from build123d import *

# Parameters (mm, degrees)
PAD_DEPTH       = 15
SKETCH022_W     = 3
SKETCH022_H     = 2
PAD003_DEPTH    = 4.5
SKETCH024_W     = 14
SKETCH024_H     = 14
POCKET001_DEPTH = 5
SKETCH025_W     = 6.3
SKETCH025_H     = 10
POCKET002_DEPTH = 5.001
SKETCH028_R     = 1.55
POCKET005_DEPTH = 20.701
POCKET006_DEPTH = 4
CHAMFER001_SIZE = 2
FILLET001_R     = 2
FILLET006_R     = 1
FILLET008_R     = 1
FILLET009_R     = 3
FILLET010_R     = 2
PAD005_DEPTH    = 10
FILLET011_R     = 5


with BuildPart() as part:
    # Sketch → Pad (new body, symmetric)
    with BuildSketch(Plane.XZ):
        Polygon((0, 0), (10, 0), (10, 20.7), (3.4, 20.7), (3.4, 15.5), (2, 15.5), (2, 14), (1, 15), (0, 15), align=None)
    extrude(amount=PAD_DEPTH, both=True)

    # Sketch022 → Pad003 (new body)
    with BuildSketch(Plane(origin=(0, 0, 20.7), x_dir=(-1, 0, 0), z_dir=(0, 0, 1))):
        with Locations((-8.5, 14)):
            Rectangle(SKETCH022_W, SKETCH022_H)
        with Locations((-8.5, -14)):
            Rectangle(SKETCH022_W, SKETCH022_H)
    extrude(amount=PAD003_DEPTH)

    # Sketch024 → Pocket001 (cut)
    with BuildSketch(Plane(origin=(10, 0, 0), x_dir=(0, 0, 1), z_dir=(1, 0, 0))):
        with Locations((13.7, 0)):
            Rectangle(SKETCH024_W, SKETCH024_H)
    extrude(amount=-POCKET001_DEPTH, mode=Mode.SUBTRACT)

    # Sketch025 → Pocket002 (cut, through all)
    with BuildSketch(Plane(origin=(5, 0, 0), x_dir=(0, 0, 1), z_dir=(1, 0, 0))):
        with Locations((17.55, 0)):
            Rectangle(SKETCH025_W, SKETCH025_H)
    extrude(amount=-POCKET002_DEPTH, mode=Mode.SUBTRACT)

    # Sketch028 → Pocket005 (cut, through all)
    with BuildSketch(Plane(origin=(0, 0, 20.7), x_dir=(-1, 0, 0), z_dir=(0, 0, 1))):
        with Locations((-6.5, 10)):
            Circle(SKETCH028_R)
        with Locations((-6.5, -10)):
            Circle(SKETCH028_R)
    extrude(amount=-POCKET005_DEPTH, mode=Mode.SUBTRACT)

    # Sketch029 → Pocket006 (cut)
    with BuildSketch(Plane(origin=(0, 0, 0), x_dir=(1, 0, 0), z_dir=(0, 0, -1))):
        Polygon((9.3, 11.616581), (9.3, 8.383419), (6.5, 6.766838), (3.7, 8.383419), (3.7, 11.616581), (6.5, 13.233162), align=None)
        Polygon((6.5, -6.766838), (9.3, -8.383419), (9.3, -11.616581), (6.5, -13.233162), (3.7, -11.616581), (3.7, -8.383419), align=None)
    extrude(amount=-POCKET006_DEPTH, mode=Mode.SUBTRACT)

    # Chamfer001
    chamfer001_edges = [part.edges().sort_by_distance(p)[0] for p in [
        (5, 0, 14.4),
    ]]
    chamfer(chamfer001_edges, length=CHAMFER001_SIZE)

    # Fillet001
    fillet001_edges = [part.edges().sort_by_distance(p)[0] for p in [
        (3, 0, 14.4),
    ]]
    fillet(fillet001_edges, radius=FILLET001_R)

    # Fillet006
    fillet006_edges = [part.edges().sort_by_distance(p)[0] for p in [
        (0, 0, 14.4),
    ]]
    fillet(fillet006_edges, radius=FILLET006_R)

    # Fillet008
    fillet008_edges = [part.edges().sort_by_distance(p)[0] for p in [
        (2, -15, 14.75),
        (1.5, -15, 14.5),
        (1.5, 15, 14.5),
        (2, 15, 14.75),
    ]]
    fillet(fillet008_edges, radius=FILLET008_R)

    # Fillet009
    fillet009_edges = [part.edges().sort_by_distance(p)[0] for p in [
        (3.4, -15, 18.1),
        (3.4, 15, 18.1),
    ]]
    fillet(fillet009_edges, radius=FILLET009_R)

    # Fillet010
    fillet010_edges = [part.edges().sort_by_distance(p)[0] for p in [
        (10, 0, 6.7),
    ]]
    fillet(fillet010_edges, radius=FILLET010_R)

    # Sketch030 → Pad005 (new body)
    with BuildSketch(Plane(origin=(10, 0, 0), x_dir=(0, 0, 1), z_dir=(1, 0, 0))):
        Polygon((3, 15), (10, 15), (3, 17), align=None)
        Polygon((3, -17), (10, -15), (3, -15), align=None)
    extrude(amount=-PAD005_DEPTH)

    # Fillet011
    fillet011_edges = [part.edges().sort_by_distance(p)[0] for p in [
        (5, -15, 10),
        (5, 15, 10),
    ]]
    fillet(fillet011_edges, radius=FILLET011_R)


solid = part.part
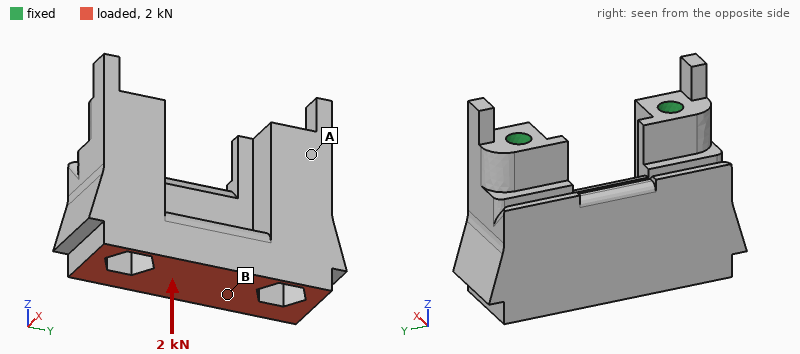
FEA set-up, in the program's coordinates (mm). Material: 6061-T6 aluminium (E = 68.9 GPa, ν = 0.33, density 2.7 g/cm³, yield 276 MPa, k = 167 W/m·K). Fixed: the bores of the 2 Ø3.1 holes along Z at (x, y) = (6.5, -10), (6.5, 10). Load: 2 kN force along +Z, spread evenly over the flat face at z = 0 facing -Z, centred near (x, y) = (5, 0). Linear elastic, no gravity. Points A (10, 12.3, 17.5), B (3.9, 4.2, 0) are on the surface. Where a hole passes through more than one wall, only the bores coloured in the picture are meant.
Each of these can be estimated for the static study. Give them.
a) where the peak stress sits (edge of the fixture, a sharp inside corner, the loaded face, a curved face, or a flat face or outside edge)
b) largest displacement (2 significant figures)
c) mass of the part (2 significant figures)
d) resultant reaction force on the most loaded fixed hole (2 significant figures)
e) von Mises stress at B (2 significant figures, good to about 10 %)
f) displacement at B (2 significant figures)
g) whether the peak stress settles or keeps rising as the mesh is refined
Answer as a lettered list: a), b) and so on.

a) edge of the fixture
b) 3.8 µm
c) 11 g
d) 1.0 kN
e) 8.7 MPa
f) 2.6 µm
g) keeps rising
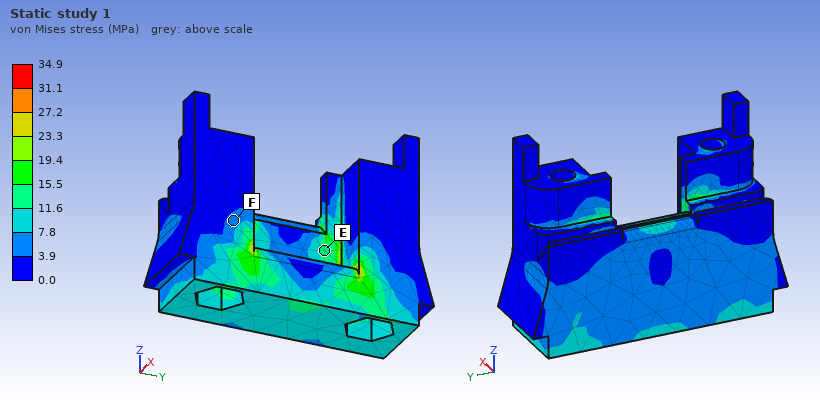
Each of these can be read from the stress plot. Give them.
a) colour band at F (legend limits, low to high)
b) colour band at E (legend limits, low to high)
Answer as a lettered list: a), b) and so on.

a) 3.9 to 7.8 MPa
b) 11.6 to 15.5 MPa
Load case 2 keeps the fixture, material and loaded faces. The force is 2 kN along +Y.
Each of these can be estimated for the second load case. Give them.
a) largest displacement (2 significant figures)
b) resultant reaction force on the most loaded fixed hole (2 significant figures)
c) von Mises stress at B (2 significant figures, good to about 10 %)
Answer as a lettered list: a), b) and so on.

a) 5.9 µm
b) 1.1 kN
c) 16 MPa
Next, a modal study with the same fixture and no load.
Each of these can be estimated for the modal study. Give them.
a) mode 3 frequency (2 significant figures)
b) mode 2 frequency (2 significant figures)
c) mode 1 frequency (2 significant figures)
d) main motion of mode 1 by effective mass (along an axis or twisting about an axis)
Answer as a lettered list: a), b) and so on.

a) 50 kHz
b) 50 kHz
c) 43 kHz
d) along X
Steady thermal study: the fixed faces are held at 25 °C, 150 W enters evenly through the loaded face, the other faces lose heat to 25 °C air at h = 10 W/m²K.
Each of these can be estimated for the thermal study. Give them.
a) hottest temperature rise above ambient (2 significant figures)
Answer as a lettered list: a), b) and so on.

a) 44 K
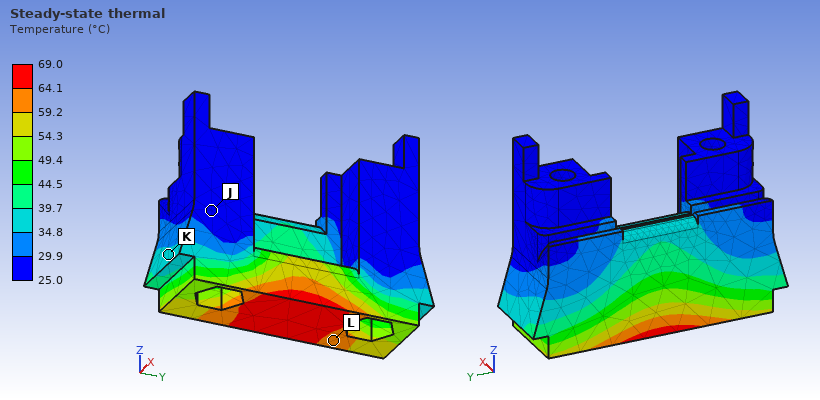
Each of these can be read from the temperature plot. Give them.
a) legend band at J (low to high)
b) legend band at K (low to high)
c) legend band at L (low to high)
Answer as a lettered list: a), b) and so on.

a) 25.0 to 29.9 °C
b) 34.8 to 39.7 °C
c) 59.2 to 64.1 °C
